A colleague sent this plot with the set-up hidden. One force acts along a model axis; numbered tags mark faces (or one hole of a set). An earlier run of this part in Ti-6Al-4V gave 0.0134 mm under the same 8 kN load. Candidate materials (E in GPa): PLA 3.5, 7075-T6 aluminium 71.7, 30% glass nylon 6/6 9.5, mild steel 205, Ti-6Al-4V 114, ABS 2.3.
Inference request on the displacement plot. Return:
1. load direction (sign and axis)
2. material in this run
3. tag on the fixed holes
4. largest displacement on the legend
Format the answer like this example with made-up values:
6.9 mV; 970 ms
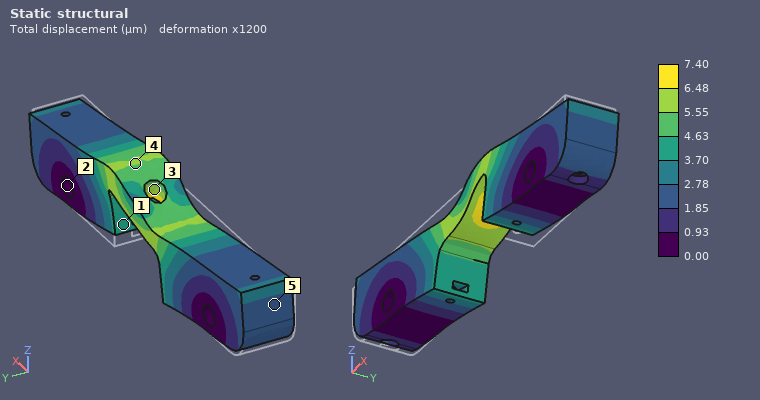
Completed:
+X; mild steel; 2; 7.40 µm
